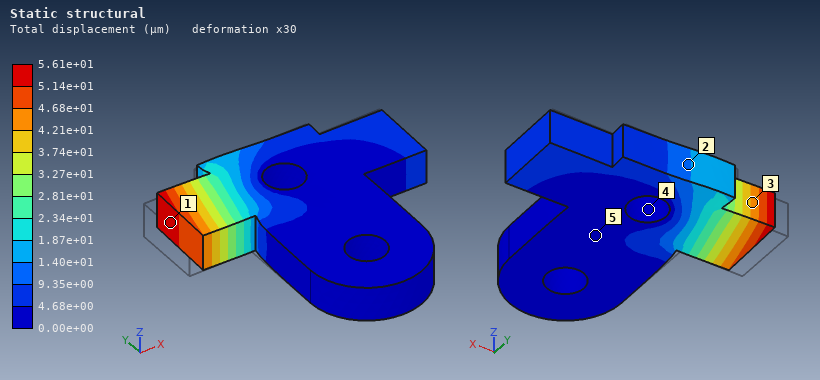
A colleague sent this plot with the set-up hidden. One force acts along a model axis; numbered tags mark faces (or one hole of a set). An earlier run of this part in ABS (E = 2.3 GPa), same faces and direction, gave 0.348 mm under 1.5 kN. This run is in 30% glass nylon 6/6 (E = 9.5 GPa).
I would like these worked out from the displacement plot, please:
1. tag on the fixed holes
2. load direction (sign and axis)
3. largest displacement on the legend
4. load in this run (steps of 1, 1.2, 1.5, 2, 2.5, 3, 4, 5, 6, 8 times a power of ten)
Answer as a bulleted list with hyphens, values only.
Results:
- 4
- +X
- 5.61e+01 µm
- 1 kN
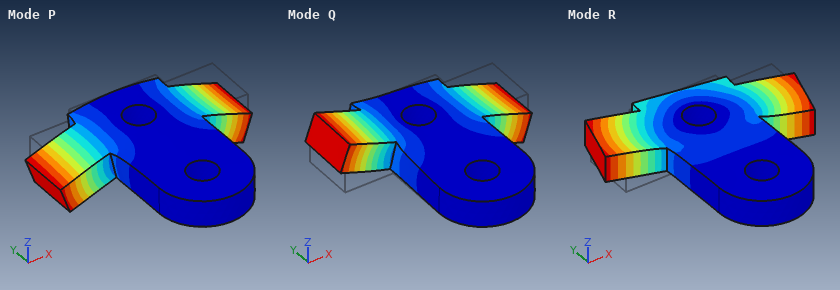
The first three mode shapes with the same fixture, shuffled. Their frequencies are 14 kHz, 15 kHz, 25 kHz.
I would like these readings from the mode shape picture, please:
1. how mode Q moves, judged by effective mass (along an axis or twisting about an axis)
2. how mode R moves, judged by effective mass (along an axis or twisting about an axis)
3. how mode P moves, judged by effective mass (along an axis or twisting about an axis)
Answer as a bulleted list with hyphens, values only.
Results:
- twisting about Y
- twisting about Z
- along Z
